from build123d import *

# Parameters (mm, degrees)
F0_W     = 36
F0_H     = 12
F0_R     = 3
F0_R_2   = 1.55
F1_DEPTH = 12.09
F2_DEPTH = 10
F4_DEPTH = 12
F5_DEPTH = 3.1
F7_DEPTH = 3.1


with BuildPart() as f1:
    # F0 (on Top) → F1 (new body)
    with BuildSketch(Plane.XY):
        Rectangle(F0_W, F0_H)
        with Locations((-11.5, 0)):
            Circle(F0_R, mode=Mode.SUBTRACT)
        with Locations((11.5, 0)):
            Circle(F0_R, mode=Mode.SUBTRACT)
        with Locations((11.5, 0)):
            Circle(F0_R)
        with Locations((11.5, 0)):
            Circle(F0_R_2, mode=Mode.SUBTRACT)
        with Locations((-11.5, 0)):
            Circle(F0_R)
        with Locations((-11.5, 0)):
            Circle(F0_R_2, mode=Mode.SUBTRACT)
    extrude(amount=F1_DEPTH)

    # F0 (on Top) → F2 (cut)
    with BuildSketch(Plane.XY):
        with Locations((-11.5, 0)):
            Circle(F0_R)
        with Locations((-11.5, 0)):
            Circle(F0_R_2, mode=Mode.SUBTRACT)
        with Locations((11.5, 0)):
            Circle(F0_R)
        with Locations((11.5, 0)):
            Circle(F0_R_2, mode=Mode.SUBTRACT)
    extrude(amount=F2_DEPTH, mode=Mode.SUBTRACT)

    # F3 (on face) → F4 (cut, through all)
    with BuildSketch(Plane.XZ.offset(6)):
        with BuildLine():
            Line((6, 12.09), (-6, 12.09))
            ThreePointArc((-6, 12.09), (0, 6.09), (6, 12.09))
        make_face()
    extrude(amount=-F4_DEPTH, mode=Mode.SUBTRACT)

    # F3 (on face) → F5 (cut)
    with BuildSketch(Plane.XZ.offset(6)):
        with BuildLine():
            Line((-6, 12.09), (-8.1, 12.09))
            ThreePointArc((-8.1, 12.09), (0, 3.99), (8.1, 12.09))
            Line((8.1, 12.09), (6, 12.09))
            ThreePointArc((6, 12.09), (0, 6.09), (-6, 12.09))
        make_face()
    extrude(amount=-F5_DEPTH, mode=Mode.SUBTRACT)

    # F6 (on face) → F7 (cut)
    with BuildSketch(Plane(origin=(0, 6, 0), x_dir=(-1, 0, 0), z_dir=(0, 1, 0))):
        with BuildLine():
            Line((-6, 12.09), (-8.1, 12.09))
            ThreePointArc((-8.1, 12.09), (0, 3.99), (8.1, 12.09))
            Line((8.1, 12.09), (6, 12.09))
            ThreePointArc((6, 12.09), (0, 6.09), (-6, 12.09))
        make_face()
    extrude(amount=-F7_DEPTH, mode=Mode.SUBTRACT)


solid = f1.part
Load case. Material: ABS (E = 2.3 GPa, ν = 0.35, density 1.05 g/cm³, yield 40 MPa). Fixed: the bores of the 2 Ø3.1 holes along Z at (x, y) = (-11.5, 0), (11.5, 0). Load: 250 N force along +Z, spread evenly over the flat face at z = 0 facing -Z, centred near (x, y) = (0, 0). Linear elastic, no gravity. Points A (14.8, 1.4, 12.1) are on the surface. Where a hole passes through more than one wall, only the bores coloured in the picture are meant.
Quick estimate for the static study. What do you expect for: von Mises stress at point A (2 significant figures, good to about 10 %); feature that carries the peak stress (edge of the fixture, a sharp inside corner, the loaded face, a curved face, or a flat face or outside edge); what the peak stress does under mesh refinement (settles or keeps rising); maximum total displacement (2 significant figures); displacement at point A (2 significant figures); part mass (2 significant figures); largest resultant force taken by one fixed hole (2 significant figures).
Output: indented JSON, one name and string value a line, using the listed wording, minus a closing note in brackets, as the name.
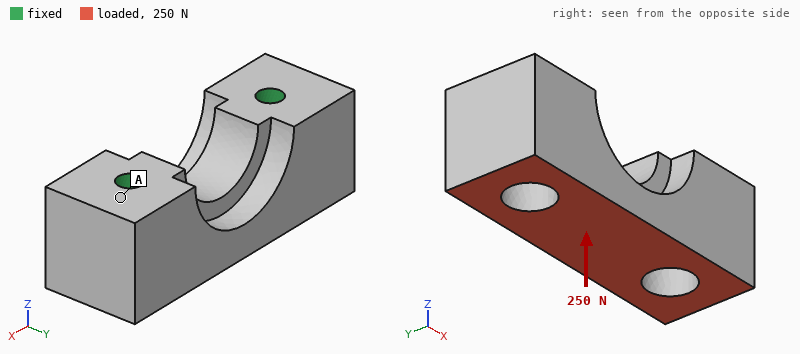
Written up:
{
  "von Mises stress at point A": "3.2 MPa",
  "feature that carries the peak stress": "edge of the fixture",
  "what the peak stress does under mesh refinement": "keeps rising",
  "maximum total displacement": "29 µm",
  "displacement at point A": "12 µm",
  "part mass": "3.8 g",
  "largest resultant force taken by one fixed hole": "130 N"
}
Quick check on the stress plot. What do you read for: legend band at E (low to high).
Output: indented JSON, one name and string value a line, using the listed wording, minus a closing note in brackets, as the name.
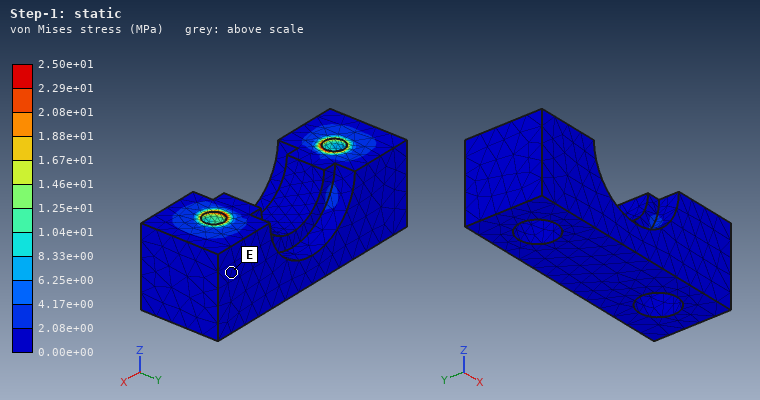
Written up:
{
  "legend band at E": "0.00e+00 to 2.08e+00 MPa"
}
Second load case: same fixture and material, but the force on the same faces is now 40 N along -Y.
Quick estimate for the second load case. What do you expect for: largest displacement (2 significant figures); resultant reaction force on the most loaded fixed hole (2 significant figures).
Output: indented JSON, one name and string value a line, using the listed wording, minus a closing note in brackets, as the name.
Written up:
{
  "largest displacement": "95 µm",
  "resultant reaction force on the most loaded fixed hole": "20 N"
}
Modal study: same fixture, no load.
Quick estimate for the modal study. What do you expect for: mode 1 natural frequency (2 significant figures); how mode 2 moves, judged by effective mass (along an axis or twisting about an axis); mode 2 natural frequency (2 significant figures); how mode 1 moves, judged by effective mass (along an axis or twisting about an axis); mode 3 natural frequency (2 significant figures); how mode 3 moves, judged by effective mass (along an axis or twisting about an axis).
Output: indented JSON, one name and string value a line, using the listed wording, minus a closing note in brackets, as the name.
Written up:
{
  "mode 1 natural frequency": "2700 Hz",
  "how mode 2 moves, judged by effective mass": "twisting about Z",
  "mode 2 natural frequency": "5000 Hz",
  "how mode 1 moves, judged by effective mass": "along Y",
  "mode 3 natural frequency": "6700 Hz",
  "how mode 3 moves, judged by effective mass": "along X"
}
